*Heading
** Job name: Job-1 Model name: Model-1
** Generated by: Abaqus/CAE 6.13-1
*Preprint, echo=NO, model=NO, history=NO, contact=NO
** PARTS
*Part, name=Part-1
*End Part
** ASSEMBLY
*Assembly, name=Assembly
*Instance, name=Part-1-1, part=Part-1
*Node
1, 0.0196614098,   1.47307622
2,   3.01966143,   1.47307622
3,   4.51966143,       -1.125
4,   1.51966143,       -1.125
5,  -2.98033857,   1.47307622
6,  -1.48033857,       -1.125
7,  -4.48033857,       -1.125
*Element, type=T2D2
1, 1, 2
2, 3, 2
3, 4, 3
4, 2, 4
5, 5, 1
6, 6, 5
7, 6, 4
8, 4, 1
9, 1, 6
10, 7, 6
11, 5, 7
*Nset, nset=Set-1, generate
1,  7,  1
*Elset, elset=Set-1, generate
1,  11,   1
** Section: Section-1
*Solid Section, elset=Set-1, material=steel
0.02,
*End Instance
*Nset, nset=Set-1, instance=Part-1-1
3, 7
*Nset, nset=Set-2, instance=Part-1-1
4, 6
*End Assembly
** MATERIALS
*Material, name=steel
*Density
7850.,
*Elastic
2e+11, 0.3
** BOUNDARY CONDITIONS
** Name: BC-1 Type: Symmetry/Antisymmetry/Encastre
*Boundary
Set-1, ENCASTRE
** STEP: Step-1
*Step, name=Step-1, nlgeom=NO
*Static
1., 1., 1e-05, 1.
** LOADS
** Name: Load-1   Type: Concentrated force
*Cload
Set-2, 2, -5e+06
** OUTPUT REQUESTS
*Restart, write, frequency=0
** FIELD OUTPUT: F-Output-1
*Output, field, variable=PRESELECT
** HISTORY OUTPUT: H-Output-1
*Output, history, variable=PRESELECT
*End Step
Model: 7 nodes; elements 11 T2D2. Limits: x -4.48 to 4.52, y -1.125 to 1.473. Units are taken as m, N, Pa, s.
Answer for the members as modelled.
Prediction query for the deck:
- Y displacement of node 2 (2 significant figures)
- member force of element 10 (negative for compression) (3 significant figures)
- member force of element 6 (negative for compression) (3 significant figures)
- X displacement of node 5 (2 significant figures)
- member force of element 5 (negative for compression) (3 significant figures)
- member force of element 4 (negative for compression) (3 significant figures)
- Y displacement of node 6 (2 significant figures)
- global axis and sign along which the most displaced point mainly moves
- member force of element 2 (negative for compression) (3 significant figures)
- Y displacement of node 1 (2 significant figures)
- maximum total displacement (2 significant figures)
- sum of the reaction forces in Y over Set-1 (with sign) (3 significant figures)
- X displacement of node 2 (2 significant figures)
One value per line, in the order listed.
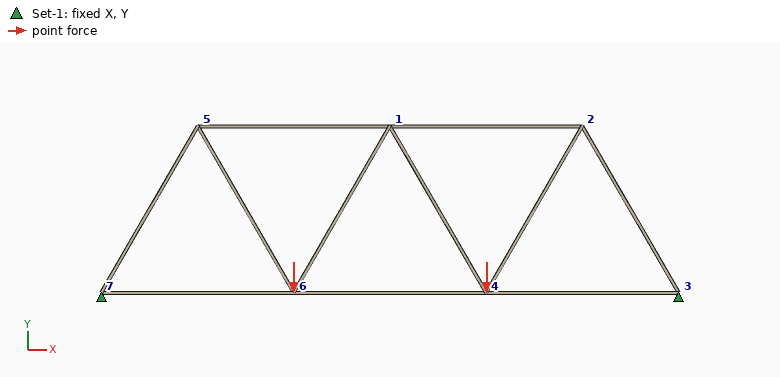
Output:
-0.0075 m
-9.62e+05 N
5.77e+06 N
0.0043 m
-5.77e+06 N
5.77e+06 N
-0.015 m
-Y
-5.77e+06 N
-0.016 m
0.016 m
1.00e+07 N
-0.0043 m
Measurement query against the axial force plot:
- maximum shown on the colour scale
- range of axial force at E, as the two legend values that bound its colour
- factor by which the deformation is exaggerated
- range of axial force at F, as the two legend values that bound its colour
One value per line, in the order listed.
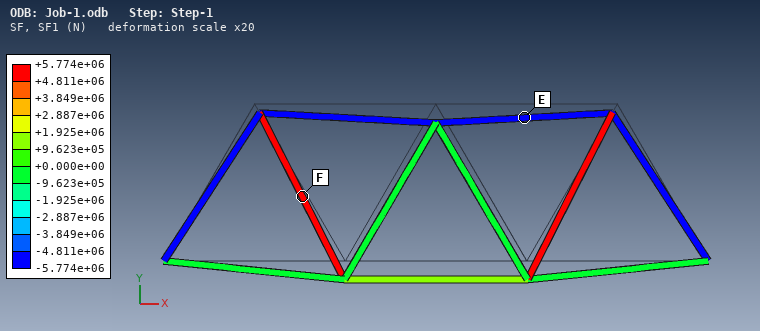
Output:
+5.774e+06 N
-5.774e+06 to -4.811e+06 N
20
+4.811e+06 to +5.774e+06 N
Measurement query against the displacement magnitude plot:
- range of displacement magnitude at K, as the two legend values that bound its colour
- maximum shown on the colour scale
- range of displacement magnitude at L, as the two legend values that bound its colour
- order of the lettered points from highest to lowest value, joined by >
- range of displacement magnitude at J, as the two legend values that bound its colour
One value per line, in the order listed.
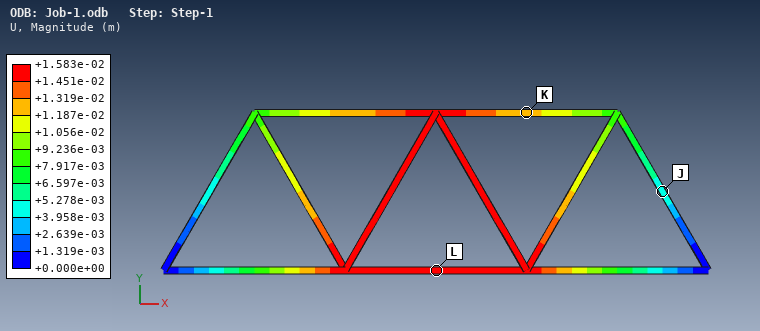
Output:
+1.187e-02 to +1.319e-02 m
+1.583e-02 m
+1.451e-02 to +1.583e-02 m
L > K > J
+3.958e-03 to +5.278e-03 m
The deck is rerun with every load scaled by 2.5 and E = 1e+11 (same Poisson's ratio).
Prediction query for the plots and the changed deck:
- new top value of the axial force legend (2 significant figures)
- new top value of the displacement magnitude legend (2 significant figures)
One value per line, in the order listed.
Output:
1.4e+07 N
0.079 m
